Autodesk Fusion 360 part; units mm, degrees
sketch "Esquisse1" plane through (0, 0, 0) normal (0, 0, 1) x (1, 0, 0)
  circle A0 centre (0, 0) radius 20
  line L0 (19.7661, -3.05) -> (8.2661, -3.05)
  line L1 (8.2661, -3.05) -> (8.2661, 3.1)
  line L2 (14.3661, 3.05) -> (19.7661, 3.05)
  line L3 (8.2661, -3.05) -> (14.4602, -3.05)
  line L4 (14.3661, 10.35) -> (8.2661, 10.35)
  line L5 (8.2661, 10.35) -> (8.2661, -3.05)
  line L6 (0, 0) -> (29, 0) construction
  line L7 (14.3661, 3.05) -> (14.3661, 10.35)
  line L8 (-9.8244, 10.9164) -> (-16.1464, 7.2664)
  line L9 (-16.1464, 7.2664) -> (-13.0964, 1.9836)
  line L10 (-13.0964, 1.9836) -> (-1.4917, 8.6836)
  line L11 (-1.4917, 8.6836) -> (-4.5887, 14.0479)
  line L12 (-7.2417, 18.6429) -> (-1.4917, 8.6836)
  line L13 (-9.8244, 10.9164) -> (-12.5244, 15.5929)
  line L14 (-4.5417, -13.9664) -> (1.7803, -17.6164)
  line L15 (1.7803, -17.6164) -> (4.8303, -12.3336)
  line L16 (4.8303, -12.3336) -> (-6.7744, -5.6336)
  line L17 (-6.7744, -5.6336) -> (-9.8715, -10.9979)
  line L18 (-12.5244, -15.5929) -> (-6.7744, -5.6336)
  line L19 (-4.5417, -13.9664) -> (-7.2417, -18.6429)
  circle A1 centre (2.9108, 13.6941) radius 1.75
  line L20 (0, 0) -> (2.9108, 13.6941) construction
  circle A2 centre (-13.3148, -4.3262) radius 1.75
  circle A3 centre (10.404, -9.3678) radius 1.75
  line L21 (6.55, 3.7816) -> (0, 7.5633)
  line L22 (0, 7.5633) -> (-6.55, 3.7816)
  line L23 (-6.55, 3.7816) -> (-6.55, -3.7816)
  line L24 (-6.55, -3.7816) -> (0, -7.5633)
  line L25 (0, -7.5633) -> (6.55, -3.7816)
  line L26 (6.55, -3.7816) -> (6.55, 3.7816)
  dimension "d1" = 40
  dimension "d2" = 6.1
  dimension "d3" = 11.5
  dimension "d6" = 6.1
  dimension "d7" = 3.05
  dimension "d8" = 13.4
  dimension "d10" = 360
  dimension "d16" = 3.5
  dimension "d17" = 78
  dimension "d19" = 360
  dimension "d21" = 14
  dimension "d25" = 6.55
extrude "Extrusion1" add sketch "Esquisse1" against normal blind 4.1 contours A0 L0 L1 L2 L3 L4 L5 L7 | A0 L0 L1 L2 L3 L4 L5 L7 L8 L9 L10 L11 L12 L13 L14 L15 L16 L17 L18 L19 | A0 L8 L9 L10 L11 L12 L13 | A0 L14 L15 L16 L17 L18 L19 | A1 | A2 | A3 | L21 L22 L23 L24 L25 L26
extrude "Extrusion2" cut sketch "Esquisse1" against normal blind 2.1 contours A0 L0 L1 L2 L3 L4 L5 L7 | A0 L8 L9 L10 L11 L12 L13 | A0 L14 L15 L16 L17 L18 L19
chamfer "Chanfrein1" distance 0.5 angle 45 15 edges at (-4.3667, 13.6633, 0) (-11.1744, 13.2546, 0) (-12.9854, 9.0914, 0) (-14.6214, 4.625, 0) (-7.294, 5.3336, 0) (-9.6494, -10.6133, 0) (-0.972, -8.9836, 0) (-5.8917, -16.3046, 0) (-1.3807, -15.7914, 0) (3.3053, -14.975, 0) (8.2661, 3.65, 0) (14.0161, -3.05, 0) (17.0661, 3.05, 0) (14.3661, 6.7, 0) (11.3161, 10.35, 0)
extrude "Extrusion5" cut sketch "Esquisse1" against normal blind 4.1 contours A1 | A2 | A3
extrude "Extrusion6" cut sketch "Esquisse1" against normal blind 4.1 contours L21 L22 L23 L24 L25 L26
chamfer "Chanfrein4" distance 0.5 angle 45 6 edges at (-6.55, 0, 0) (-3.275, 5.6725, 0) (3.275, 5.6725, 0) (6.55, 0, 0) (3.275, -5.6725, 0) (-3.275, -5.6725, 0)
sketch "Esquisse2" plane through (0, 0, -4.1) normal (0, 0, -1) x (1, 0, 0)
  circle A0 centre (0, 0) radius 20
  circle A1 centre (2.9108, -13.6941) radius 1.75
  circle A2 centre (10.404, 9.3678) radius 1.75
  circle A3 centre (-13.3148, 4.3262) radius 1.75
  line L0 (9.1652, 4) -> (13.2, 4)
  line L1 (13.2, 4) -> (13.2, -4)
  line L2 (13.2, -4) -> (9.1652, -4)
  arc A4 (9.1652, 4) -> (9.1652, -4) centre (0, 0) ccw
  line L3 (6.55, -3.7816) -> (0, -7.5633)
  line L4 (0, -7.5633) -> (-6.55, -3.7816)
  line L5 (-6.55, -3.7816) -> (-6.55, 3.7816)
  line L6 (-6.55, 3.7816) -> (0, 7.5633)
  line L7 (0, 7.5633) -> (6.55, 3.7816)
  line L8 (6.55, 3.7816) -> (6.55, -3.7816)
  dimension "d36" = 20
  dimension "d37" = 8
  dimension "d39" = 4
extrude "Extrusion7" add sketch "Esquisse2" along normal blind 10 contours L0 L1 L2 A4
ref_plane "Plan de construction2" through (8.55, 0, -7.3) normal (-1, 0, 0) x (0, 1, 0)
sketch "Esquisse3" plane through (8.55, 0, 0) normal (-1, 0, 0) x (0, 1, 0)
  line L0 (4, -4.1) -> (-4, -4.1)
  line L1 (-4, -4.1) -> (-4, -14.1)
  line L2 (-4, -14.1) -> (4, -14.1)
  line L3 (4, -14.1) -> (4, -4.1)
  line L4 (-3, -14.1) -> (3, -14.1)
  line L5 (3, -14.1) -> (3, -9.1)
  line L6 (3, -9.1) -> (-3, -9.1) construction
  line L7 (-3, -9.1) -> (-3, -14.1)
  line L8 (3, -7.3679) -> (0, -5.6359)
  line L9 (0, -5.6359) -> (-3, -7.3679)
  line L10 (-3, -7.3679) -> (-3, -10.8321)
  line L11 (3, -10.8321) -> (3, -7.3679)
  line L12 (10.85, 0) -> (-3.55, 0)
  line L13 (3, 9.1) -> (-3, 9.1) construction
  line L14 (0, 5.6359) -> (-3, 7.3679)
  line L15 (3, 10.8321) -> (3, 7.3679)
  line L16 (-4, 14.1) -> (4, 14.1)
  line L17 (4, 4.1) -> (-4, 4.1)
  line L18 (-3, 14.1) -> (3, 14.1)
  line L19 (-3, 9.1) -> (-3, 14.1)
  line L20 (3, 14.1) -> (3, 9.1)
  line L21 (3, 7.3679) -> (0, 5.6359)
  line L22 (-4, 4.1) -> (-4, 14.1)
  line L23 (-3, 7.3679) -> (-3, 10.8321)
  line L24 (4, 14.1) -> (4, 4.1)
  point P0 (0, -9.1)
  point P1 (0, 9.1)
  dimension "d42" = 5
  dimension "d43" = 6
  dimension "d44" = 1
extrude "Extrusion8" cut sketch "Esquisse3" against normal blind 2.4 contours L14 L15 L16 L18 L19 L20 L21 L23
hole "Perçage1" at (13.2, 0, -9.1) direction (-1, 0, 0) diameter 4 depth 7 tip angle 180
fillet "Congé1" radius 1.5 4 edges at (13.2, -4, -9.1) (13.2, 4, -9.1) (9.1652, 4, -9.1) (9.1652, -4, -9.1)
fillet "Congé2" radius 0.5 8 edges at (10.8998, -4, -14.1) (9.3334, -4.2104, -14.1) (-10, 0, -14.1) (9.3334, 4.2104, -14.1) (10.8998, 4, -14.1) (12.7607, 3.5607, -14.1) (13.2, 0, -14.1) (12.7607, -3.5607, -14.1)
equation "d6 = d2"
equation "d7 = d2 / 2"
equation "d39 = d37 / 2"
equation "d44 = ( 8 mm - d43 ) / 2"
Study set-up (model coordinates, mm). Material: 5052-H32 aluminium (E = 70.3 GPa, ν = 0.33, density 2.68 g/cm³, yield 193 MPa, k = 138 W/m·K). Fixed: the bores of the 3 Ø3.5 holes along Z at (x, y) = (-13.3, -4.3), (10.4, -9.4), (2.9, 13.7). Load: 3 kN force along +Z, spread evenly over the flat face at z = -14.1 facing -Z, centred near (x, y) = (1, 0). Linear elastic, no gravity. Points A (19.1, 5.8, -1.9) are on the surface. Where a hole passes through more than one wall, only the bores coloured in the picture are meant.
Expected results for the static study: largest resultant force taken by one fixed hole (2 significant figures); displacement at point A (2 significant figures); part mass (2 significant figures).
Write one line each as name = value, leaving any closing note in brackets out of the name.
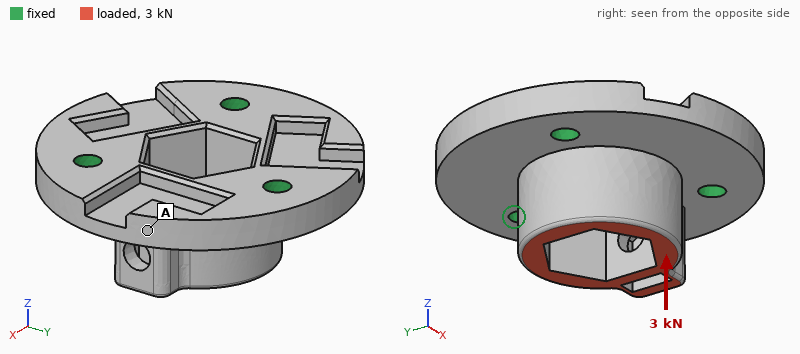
largest resultant force taken by one fixed hole = 1.2 kN
displacement at point A = 9.3 µm
part mass = 15 g
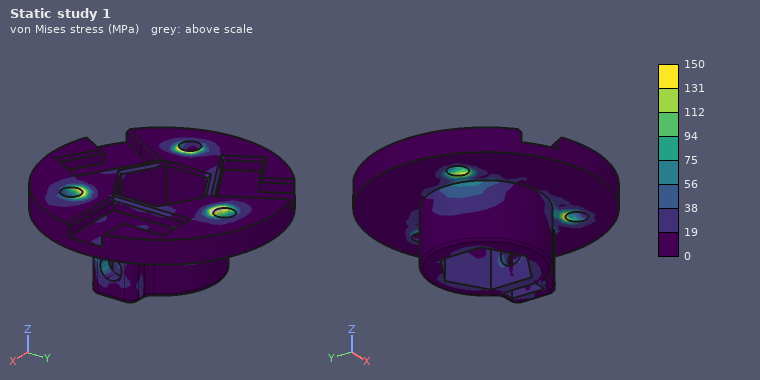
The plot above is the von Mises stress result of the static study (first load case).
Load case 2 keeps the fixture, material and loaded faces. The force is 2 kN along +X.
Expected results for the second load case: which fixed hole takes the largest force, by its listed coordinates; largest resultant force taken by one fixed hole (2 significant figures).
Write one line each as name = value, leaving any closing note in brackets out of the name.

which fixed hole takes the largest force, by its listed coordinates = (-13.3, -4.3)
largest resultant force taken by one fixed hole = 1.3 kN
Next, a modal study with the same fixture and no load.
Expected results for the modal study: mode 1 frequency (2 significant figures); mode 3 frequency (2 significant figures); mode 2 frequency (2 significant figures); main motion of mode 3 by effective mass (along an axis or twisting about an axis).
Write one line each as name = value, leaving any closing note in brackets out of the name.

mode 1 frequency = 18 kHz
mode 3 frequency = 21 kHz
mode 2 frequency = 19 kHz
main motion of mode 3 by effective mass = along Z
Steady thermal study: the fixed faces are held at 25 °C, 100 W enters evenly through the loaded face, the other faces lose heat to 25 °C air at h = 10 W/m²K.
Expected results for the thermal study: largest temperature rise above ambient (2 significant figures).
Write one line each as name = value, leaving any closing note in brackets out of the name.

largest temperature rise above ambient = 77 K
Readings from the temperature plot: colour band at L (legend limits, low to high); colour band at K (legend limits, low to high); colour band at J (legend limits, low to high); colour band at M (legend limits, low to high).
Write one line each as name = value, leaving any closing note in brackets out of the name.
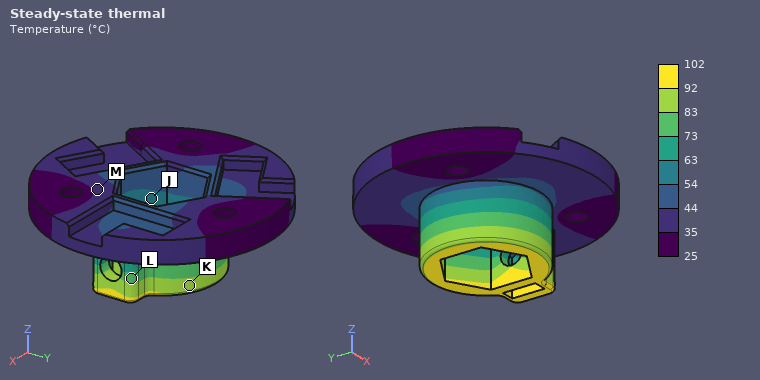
colour band at L = 73 to 83 °C
colour band at K = 83 to 92 °C
colour band at J = 54 to 63 °C
colour band at M = 35 to 44 °C
